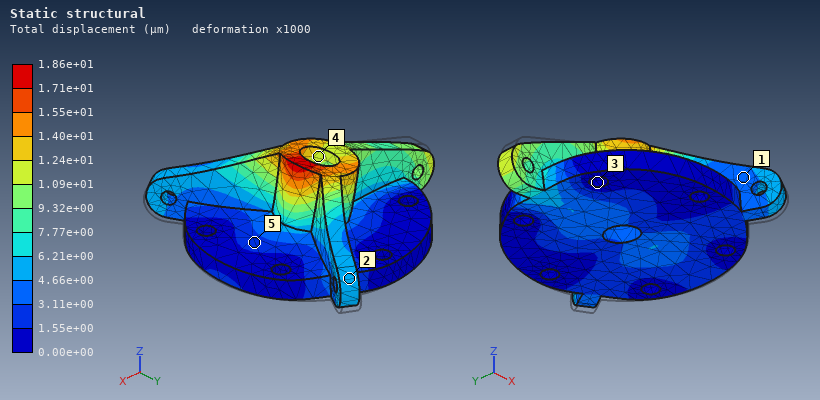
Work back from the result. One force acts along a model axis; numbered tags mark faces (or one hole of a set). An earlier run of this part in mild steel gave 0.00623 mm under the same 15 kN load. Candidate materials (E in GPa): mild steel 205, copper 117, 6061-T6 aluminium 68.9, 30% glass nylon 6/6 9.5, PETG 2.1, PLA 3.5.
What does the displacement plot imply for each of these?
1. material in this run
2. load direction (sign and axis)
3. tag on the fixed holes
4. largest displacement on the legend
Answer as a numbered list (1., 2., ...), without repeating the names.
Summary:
1. 6061-T6 aluminium
2. -X
3. 3
4. 1.86e+01 µm
